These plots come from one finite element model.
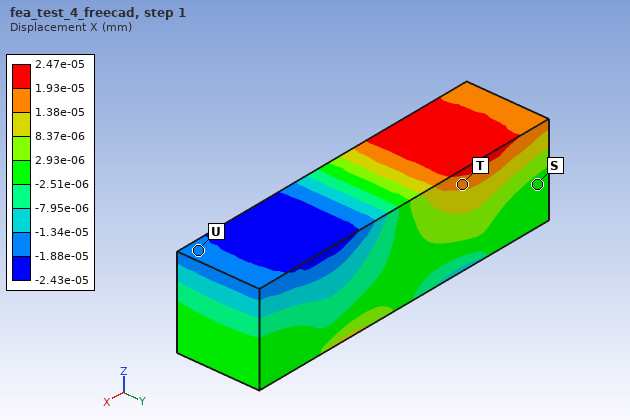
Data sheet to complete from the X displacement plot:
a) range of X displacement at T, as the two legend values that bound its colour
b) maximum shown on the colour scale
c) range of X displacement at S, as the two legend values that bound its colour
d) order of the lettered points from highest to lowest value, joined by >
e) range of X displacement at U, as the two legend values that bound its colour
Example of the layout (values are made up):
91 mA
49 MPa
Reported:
1.38e-05 to 1.93e-05 mm
2.47e-05 mm
-2.51e-06 to 2.93e-06 mm
T > S > U
-1.88e-05 to -1.34e-05 mm
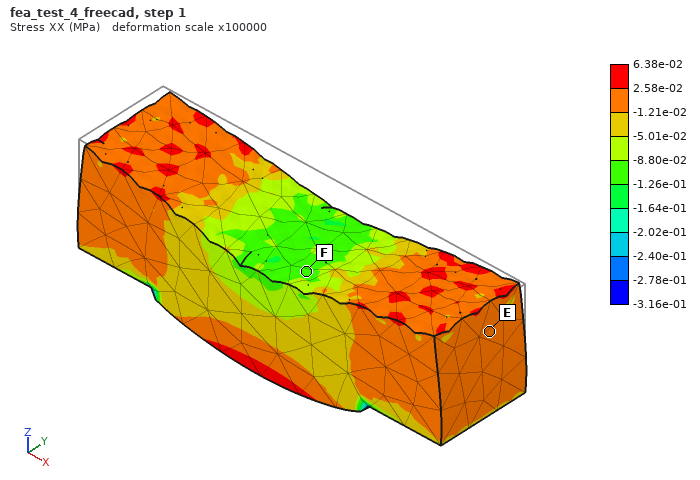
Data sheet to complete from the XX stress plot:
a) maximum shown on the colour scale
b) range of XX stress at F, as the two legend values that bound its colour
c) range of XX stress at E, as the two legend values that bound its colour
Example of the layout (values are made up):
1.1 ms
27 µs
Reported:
6.38e-02 MPa
-1.26e-01 to -8.80e-02 MPa
-1.21e-02 to 2.58e-02 MPa
